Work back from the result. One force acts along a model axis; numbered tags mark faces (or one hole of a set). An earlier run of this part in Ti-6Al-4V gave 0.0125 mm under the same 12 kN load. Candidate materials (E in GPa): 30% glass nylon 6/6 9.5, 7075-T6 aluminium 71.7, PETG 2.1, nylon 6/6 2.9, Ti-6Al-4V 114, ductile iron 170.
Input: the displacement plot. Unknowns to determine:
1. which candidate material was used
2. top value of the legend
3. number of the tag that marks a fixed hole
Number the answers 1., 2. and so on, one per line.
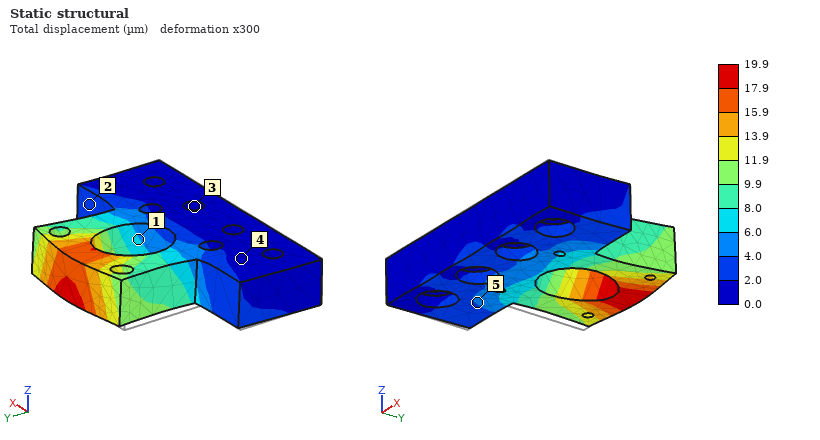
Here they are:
1. 7075-T6 aluminium
2. 19.9 µm
3. 3
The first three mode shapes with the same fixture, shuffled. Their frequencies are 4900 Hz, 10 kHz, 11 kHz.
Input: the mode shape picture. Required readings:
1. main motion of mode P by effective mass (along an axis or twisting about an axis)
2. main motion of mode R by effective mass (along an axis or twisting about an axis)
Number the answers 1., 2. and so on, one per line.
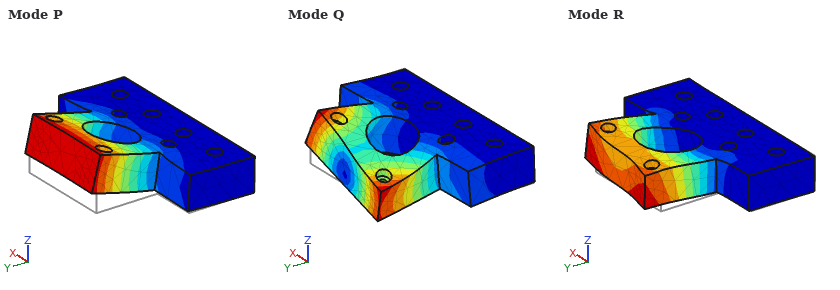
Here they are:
1. along Z
2. along X
